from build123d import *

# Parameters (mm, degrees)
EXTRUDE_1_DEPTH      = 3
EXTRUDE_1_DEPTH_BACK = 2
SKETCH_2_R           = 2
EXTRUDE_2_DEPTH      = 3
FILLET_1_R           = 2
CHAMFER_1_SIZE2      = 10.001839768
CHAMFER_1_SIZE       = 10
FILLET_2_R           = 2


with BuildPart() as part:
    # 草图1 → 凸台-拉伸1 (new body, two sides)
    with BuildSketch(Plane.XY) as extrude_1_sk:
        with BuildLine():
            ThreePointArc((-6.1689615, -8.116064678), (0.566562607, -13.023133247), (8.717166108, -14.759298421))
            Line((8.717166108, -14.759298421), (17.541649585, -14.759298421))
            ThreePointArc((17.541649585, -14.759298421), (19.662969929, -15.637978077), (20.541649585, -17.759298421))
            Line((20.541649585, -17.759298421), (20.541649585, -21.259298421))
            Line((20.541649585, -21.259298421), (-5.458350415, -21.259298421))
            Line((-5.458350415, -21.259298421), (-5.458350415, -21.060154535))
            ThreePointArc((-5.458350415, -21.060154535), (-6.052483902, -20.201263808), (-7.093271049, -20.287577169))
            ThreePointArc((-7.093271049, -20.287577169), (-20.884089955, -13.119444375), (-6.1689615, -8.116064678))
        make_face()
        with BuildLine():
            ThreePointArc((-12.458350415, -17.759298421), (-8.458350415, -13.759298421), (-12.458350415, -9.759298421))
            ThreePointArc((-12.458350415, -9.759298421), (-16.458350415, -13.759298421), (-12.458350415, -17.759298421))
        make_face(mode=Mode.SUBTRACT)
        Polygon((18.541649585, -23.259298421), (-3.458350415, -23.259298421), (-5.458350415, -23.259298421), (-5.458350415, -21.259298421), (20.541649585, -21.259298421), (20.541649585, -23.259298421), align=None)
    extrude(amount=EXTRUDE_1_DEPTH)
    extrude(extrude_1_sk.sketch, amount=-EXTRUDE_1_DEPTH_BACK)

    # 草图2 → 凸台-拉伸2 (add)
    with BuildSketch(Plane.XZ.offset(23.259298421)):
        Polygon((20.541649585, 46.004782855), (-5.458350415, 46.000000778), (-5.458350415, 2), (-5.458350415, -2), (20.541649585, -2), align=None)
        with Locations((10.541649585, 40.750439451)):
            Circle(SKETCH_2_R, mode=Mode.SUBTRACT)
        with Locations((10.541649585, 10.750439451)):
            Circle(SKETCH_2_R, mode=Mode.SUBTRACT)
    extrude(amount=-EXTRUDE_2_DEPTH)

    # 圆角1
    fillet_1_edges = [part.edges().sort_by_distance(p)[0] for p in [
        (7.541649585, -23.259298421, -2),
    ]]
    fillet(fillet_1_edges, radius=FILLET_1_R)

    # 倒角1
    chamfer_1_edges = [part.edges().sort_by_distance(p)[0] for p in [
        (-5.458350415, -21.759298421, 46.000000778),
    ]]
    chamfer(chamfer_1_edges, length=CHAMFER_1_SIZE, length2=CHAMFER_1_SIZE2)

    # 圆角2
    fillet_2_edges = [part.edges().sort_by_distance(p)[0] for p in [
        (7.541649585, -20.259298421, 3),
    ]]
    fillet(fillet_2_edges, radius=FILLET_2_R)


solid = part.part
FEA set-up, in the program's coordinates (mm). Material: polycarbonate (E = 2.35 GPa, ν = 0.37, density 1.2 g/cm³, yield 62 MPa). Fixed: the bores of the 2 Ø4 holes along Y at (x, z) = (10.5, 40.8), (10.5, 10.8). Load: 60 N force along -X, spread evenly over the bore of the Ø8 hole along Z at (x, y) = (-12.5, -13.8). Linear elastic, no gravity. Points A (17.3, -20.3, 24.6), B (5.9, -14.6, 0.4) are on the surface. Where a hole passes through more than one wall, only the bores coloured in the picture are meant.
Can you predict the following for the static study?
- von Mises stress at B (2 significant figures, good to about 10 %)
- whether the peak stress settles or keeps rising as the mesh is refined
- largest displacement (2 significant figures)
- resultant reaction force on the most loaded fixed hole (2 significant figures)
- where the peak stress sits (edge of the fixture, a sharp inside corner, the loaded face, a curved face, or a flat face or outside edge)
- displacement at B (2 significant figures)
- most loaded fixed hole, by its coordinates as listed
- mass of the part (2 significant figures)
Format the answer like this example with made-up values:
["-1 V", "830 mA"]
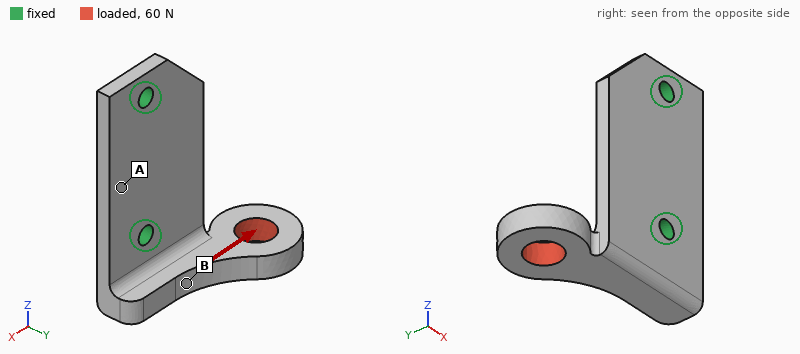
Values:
["5.7 MPa", "keeps rising", "0.63 mm", "76 N", "edge of the fixture", "0.15 mm", "(10.5, 10.8)", "6.2 g"]
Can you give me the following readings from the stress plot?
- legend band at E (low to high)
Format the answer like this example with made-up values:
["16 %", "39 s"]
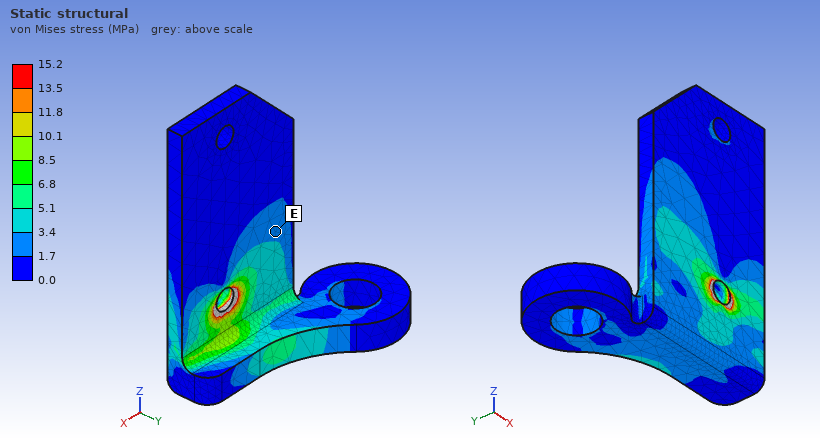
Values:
["1.7 to 3.4 MPa"]
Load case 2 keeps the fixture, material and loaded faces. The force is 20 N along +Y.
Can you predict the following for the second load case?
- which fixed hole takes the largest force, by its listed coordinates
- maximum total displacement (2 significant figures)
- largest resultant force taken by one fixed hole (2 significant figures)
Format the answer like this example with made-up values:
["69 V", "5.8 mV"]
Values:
["(10.5, 10.8)", "0.70 mm", "22 N"]
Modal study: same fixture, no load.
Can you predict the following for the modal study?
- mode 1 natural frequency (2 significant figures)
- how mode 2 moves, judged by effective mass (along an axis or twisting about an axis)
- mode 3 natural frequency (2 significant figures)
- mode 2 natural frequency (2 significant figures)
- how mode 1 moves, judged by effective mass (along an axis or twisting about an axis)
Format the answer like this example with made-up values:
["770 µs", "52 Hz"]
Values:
["820 Hz", "along Z", "2500 Hz", "1400 Hz", "along Y"]
